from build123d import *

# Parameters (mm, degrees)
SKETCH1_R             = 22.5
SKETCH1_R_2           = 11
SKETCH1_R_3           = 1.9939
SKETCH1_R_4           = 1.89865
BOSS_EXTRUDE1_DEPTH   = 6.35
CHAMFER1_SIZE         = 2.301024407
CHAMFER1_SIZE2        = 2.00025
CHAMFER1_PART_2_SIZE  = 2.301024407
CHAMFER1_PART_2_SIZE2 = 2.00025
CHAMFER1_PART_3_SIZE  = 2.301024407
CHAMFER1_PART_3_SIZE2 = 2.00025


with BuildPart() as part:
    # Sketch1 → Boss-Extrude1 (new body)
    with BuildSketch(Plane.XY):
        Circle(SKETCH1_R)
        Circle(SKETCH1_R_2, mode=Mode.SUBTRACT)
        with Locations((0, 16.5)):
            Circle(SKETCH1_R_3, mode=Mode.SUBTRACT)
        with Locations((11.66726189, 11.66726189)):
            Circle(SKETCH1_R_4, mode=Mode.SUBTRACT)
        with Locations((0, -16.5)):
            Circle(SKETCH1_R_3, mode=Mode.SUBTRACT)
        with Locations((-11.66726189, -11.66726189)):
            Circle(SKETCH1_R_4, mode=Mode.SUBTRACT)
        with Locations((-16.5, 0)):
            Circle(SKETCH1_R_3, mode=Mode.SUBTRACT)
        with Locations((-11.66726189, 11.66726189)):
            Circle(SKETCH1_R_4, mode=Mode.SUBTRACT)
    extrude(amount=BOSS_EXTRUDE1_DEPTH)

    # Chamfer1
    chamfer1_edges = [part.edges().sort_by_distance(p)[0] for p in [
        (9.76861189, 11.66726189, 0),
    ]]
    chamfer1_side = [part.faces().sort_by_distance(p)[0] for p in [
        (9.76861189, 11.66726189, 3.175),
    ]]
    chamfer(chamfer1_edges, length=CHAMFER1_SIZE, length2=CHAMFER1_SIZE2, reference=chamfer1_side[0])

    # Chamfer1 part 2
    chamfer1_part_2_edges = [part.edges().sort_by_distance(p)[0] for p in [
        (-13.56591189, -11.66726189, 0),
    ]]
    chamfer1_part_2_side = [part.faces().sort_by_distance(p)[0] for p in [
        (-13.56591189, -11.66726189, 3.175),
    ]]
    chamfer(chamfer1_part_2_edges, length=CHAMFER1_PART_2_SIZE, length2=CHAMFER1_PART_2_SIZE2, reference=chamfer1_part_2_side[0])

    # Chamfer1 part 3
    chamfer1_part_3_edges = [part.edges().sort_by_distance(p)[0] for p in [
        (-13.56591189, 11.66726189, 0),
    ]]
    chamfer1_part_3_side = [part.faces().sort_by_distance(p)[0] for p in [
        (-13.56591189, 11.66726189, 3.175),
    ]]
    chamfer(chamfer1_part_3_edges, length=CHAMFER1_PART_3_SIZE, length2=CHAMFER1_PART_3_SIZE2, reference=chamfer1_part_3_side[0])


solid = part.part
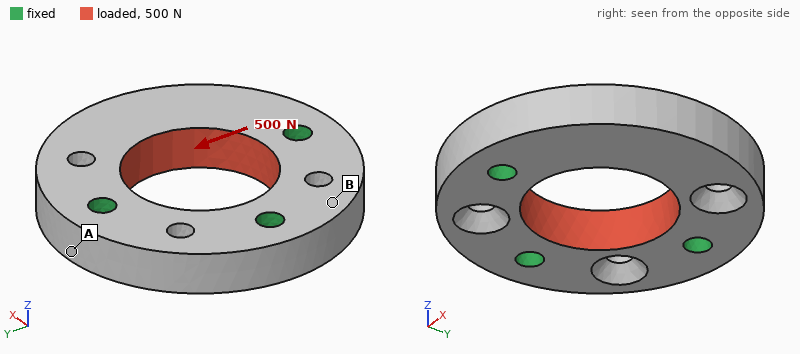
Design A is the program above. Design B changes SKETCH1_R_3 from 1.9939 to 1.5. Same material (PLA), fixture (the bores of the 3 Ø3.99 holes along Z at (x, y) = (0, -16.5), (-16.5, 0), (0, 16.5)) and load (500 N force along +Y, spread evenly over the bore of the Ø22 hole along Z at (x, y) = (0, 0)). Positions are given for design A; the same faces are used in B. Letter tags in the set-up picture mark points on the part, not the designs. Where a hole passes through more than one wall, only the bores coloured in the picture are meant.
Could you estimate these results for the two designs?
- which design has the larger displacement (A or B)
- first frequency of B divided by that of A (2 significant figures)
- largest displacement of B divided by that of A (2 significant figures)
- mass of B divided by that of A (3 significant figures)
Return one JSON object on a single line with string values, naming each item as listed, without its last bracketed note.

{"which design has the larger displacement": "B", "first frequency of B divided by that of A": "0.94", "largest displacement of B divided by that of A": "1.1", "mass of B divided by that of A": "1.01"}
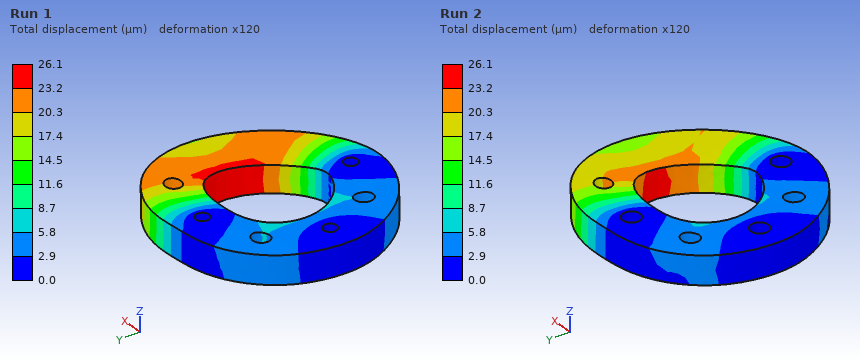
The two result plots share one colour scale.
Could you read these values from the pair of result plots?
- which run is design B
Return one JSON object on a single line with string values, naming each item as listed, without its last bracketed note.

{"which run is design B": "Run 1"}
